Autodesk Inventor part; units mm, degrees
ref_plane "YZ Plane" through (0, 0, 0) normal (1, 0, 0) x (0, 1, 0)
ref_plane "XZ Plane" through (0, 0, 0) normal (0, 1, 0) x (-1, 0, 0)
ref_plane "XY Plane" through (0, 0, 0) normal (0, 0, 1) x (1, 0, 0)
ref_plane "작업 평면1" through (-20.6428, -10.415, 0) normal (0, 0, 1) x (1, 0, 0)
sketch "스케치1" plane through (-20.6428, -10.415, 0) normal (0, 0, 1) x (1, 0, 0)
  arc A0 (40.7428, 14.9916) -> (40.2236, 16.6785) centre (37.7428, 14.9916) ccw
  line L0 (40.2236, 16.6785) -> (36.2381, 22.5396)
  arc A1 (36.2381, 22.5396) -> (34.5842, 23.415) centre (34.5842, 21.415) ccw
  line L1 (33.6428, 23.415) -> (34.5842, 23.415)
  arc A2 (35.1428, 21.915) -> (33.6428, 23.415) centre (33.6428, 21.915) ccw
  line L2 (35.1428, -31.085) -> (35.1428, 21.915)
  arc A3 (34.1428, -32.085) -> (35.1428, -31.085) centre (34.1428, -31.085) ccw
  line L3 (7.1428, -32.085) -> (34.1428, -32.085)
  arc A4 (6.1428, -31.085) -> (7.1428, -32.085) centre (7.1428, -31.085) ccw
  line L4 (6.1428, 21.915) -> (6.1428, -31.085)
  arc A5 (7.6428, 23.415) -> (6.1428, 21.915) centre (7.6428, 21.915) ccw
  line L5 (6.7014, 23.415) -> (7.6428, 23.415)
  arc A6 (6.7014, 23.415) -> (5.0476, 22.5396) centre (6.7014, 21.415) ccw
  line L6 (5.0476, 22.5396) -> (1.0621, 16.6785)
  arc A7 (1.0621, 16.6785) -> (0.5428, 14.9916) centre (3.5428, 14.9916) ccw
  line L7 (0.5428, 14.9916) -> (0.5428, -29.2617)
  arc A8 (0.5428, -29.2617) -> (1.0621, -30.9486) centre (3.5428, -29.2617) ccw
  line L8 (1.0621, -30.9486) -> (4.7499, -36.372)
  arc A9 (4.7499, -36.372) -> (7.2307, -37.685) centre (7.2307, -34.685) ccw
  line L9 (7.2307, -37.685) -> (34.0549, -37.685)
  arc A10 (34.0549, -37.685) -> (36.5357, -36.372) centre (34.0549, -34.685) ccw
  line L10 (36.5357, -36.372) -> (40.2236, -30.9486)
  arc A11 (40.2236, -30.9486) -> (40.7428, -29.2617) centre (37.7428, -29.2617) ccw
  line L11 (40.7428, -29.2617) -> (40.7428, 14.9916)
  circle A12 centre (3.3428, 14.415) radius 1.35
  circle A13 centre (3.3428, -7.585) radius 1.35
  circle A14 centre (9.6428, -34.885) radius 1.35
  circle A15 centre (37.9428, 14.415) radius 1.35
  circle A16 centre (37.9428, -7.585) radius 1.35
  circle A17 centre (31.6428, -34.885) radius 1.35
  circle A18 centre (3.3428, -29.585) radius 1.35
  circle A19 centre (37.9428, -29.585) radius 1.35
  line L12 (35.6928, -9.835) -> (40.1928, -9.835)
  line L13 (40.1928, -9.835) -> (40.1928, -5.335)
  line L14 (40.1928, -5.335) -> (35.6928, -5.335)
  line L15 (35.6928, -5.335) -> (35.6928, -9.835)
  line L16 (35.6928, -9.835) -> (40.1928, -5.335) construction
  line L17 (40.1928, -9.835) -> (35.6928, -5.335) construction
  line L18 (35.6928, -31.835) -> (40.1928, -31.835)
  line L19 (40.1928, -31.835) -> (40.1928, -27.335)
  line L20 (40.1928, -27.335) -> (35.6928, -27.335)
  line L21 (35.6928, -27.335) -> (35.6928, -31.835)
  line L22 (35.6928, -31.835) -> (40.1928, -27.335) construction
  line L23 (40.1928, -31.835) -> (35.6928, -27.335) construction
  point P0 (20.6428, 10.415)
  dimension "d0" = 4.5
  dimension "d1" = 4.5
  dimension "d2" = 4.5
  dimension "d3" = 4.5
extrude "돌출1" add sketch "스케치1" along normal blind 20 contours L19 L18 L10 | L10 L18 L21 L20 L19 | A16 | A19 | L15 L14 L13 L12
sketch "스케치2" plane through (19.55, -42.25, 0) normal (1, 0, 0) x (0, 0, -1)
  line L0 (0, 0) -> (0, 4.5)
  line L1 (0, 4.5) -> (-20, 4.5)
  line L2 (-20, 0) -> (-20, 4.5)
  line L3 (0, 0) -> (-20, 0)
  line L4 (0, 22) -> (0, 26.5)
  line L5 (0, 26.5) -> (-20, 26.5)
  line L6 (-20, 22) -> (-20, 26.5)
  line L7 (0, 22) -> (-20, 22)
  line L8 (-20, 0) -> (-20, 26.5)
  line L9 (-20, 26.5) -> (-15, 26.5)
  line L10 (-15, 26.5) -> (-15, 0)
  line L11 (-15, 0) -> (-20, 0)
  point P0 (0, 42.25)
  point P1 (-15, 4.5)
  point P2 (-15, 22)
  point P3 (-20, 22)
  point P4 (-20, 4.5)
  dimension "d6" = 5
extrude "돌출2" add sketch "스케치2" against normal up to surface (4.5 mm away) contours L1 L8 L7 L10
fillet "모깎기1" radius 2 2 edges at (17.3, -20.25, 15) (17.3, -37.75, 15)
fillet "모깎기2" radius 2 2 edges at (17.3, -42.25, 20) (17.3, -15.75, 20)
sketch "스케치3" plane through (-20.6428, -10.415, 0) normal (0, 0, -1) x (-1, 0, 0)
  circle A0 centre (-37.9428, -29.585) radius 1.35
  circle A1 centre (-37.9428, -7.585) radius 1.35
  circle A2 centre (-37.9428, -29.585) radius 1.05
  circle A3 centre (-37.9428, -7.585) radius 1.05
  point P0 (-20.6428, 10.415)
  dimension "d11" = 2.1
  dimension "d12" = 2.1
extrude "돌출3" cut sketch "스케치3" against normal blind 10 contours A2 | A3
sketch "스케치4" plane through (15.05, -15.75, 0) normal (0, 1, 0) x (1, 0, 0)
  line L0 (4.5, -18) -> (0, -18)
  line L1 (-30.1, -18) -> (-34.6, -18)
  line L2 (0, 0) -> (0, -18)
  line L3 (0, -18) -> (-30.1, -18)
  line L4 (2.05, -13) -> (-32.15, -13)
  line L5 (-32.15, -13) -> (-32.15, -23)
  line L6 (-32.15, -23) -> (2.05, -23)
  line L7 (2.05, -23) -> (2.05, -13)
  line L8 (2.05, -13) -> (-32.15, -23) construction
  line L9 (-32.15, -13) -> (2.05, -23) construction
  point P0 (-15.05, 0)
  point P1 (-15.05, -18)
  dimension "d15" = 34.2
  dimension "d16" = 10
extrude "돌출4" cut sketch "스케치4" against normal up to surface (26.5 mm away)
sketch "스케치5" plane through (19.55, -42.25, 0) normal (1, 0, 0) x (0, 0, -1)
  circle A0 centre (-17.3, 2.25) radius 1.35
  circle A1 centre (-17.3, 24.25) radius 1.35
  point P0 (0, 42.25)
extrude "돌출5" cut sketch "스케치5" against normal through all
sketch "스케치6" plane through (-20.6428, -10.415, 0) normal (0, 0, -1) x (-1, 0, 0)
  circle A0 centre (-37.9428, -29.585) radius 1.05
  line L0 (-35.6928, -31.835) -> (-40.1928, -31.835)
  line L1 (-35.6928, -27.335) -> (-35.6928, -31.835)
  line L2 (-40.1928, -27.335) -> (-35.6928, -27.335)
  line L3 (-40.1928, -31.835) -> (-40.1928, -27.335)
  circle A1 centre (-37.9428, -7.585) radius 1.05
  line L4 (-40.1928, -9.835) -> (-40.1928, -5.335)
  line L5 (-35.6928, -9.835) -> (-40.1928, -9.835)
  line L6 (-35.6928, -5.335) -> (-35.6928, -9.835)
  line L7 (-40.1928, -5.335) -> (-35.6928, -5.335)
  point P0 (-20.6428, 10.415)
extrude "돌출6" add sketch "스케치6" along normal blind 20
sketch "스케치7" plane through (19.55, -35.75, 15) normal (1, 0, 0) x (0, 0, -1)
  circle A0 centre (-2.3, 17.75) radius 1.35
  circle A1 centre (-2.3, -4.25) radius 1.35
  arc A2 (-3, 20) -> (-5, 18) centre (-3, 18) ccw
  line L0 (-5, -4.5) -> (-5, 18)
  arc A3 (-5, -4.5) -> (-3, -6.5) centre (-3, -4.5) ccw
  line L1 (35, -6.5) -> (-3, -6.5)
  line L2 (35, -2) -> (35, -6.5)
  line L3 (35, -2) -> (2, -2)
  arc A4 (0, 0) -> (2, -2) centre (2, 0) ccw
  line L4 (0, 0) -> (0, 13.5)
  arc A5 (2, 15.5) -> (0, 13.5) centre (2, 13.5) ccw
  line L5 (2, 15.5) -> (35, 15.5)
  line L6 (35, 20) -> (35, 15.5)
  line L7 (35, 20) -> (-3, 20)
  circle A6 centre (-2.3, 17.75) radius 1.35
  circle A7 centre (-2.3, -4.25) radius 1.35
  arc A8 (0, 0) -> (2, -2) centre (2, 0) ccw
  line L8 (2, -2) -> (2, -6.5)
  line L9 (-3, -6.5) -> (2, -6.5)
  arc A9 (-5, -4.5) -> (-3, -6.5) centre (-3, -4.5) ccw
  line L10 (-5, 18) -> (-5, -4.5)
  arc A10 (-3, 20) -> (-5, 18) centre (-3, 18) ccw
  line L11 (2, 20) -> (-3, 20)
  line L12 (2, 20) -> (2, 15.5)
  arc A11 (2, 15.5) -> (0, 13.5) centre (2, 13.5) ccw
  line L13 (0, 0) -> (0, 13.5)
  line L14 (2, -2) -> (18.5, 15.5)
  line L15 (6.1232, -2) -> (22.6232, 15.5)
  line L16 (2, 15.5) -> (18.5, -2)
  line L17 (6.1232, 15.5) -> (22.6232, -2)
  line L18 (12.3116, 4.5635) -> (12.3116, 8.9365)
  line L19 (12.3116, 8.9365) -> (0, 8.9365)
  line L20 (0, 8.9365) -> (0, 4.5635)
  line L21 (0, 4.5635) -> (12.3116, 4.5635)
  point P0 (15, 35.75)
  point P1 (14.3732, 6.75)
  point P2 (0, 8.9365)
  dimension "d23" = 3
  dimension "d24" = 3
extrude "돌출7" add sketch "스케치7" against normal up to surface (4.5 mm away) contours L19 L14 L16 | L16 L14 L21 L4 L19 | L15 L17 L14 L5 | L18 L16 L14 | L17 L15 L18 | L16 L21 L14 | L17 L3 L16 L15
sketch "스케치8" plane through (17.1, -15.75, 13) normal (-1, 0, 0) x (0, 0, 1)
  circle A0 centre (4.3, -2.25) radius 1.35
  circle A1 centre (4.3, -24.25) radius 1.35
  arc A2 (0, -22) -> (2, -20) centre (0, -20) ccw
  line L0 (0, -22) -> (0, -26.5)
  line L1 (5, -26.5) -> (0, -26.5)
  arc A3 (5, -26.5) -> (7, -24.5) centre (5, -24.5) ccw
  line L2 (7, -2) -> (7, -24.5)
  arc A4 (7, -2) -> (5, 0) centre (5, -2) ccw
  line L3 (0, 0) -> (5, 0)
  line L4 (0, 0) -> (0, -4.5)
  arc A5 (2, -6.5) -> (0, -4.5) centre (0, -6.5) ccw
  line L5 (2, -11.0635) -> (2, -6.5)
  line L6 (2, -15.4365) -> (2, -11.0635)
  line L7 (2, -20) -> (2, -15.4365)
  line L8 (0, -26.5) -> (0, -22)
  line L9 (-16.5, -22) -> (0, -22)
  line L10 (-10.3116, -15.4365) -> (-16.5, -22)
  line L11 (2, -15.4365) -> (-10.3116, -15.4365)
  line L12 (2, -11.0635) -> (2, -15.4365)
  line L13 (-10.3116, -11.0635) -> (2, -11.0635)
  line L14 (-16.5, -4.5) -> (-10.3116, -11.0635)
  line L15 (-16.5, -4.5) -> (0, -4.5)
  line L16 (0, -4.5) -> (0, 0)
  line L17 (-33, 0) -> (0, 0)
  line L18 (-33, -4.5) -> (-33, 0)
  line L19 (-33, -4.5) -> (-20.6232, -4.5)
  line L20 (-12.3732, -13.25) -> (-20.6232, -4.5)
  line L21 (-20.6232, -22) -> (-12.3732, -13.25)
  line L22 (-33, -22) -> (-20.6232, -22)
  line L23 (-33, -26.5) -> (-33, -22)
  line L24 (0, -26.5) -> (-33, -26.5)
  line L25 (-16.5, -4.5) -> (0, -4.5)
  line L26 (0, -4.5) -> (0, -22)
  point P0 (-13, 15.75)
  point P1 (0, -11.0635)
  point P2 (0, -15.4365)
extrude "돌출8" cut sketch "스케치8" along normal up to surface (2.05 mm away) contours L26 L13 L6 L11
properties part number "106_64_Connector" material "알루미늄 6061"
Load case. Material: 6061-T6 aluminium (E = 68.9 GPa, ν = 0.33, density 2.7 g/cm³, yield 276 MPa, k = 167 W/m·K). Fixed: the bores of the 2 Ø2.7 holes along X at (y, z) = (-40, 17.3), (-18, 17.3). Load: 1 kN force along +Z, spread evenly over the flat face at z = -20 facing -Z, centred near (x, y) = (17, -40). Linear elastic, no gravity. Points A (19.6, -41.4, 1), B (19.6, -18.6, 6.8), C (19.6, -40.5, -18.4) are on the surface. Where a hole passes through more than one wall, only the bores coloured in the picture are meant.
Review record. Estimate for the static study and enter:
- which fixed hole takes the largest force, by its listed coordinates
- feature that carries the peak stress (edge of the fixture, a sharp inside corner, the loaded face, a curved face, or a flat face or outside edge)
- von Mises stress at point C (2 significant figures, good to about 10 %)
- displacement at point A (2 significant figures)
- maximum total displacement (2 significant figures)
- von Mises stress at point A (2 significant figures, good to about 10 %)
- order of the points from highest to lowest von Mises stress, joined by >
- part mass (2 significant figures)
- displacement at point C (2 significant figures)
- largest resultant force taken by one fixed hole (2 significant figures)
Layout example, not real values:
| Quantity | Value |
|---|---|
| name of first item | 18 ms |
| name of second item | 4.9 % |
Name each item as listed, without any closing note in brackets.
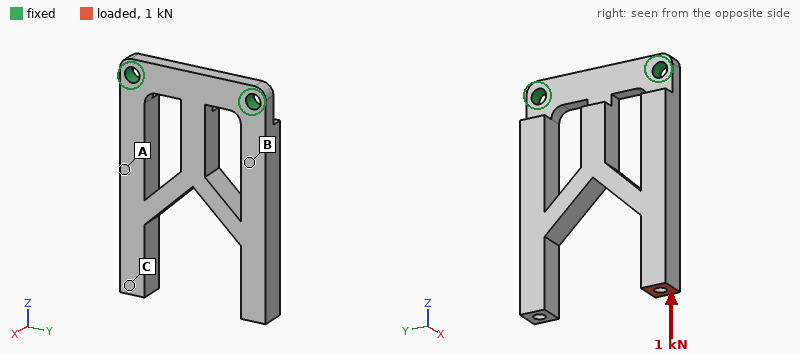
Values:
| Quantity | Value |
|---|---|
| which fixed hole takes the largest force, by its listed coordinates | (-40, 17.3) |
| feature that carries the peak stress | a flat face or outside edge |
| von Mises stress at point C | 60 MPa |
| displacement at point A | 0.081 mm |
| maximum total displacement | 0.20 mm |
| von Mises stress at point A | 74 MPa |
| order of the points from highest to lowest von Mises stress, joined by > | A > C > B |
| part mass | 5.4 g |
| displacement at point C | 0.19 mm |
| largest resultant force taken by one fixed hole | 990 N |
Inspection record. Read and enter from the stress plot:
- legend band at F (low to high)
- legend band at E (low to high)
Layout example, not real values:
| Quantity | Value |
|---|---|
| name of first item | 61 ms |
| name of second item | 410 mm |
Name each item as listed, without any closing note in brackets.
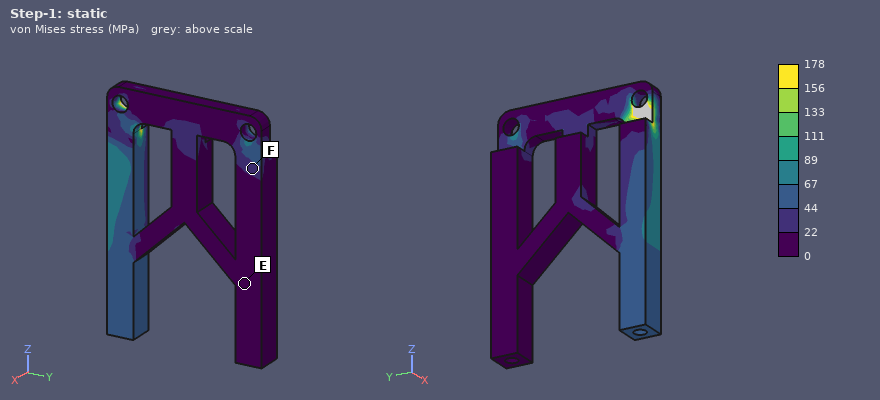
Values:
| Quantity | Value |
|---|---|
| legend band at F | 22 to 44 MPa |
| legend band at E | 0 to 22 MPa |
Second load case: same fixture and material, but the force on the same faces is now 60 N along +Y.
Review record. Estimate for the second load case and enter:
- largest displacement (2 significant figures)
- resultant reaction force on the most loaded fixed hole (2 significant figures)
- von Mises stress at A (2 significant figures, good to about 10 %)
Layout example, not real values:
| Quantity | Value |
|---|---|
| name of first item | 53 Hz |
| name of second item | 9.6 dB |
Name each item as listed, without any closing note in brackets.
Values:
| Quantity | Value |
|---|---|
| largest displacement | 72 µm |
| resultant reaction force on the most loaded fixed hole | 110 N |
| von Mises stress at A | 19 MPa |
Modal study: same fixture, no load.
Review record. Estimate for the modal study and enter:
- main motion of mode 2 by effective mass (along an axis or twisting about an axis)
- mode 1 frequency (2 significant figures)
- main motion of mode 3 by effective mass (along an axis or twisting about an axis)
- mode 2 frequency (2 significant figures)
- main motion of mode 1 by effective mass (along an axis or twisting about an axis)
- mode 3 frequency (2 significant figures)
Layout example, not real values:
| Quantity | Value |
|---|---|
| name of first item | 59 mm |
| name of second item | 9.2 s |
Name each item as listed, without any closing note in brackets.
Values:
| Quantity | Value |
|---|---|
| main motion of mode 2 by effective mass | twisting about Z |
| mode 1 frequency | 1800 Hz |
| main motion of mode 3 by effective mass | along Y |
| mode 2 frequency | 3500 Hz |
| main motion of mode 1 by effective mass | along X |
| mode 3 frequency | 6400 Hz |
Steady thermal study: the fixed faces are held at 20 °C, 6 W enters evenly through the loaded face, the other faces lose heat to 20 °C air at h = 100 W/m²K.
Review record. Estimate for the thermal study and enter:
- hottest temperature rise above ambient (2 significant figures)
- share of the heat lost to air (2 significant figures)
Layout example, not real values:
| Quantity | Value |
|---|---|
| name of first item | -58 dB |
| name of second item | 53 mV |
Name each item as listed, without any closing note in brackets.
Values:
| Quantity | Value |
|---|---|
| hottest temperature rise above ambient | 47 K |
| share of the heat lost to air | 40 % |
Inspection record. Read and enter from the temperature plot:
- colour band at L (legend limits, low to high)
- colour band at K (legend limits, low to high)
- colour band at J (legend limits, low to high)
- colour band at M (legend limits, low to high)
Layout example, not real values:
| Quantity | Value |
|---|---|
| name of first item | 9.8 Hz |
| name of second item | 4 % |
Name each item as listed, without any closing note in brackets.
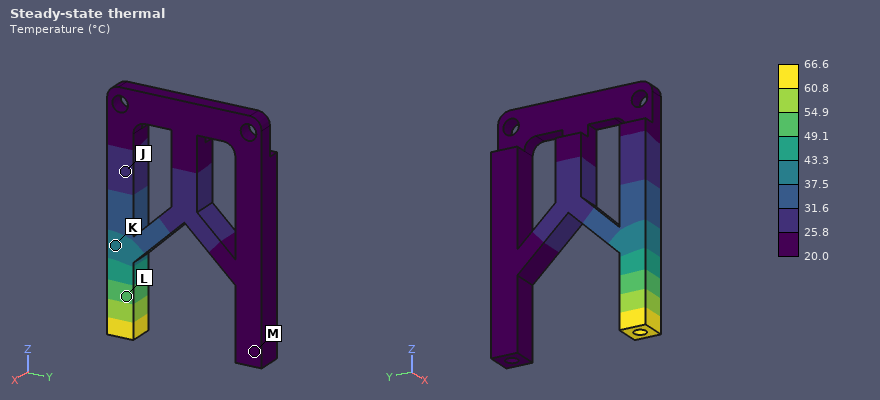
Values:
| Quantity | Value |
|---|---|
| colour band at L | 49.1 to 54.9 °C |
| colour band at K | 37.5 to 43.3 °C |
| colour band at J | 25.8 to 31.6 °C |
| colour band at M | 20.0 to 25.8 °C |
